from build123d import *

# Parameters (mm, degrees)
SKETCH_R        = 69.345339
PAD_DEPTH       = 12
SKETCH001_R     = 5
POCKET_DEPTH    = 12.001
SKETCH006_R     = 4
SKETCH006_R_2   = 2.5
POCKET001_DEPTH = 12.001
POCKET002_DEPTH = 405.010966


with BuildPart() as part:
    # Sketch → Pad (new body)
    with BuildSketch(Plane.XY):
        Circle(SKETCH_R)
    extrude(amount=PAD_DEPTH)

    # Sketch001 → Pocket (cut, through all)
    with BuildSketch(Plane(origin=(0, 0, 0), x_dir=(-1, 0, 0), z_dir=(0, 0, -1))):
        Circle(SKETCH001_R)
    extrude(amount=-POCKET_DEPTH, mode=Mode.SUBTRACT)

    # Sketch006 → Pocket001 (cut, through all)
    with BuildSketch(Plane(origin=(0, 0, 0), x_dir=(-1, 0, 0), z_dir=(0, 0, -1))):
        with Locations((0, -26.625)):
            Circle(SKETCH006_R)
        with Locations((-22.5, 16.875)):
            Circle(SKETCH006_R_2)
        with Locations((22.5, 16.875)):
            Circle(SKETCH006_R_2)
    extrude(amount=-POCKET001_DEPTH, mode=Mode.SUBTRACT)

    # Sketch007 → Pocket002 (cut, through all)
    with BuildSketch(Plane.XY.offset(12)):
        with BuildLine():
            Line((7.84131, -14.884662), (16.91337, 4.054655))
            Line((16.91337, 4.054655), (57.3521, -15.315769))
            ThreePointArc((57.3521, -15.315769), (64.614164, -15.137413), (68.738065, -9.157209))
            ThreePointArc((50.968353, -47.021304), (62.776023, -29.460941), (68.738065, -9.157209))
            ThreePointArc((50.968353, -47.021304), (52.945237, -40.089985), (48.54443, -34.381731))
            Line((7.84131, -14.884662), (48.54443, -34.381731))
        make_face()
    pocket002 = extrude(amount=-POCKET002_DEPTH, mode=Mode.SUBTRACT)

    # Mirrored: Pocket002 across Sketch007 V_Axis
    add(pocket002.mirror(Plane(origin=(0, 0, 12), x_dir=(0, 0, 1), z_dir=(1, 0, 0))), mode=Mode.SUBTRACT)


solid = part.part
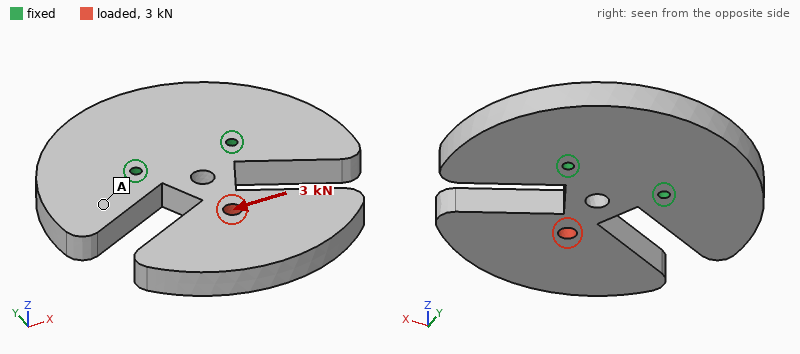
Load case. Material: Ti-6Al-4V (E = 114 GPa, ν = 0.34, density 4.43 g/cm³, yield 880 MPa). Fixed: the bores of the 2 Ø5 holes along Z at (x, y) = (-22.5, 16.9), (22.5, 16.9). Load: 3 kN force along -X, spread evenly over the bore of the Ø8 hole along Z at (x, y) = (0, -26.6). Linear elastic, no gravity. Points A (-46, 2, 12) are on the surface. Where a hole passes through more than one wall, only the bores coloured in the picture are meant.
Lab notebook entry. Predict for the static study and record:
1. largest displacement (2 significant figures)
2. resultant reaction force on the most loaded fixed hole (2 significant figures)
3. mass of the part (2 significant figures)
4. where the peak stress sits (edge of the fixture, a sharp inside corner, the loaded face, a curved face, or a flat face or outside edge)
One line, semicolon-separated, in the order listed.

0.10 mm; 3.3 kN; 660 g; a flat face or outside edge
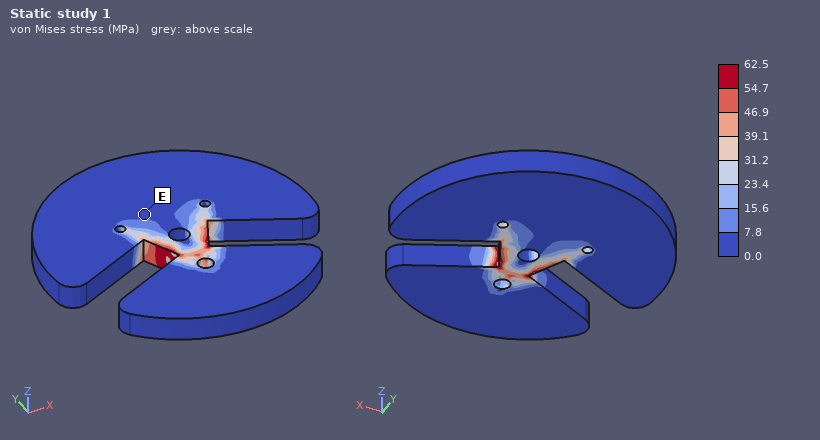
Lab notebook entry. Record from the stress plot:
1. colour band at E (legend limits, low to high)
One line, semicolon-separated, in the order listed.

0.0 to 7.8 MPa
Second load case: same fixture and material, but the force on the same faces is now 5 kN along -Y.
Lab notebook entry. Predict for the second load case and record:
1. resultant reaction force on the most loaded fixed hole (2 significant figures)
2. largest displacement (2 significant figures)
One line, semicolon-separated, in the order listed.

2.6 kN; 11 µm
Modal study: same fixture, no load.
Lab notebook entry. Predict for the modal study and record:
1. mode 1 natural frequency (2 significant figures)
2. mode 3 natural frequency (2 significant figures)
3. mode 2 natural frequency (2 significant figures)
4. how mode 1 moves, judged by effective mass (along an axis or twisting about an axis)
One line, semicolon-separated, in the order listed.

710 Hz; 1300 Hz; 1300 Hz; along Z
